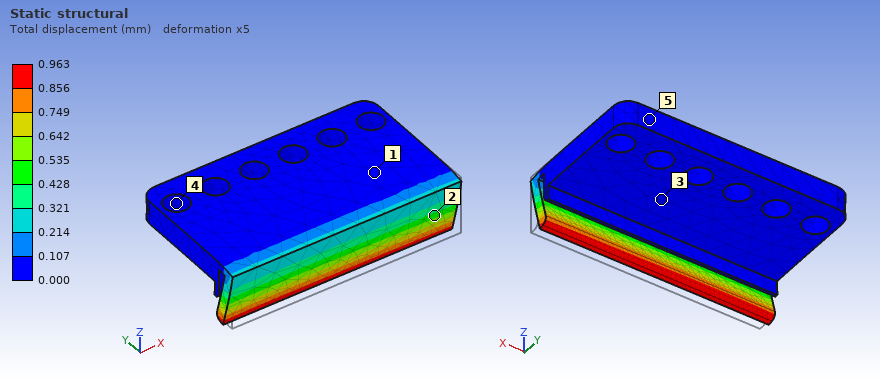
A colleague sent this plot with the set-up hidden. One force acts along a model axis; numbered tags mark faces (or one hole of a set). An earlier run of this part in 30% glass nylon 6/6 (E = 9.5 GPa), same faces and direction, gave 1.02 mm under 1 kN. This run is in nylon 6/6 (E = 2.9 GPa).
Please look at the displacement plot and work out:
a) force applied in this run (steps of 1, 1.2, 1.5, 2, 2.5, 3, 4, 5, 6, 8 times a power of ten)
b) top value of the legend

300 N
0.963 mm
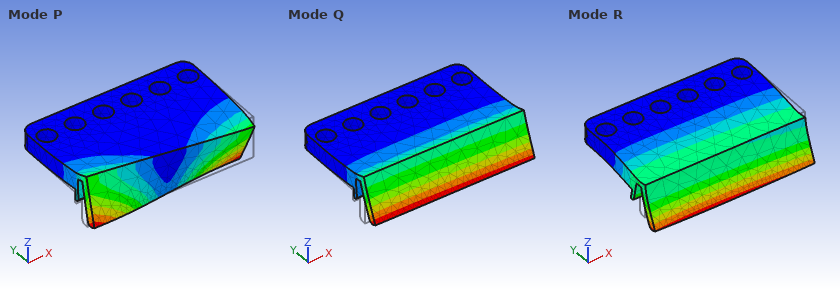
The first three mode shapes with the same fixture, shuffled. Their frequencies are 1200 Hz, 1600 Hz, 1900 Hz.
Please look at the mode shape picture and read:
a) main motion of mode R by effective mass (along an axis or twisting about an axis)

along Z
